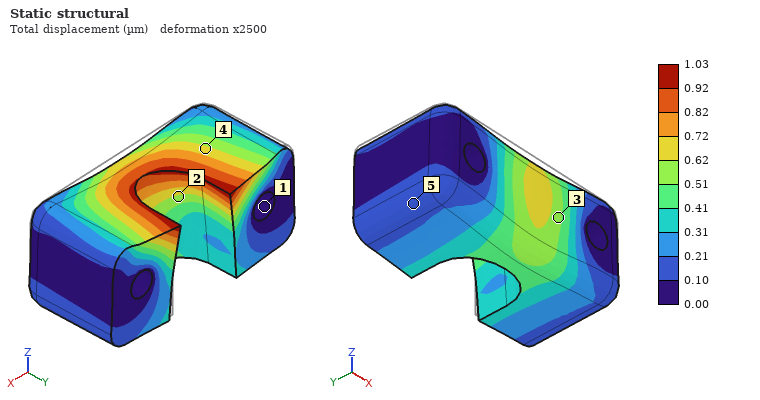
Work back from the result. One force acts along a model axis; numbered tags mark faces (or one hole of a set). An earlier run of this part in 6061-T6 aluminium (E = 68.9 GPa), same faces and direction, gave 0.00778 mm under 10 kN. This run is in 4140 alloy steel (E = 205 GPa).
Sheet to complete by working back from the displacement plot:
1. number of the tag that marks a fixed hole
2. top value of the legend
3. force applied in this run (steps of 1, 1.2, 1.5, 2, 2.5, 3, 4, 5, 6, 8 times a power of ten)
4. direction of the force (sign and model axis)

1
1.03 µm
4 kN
-Z
